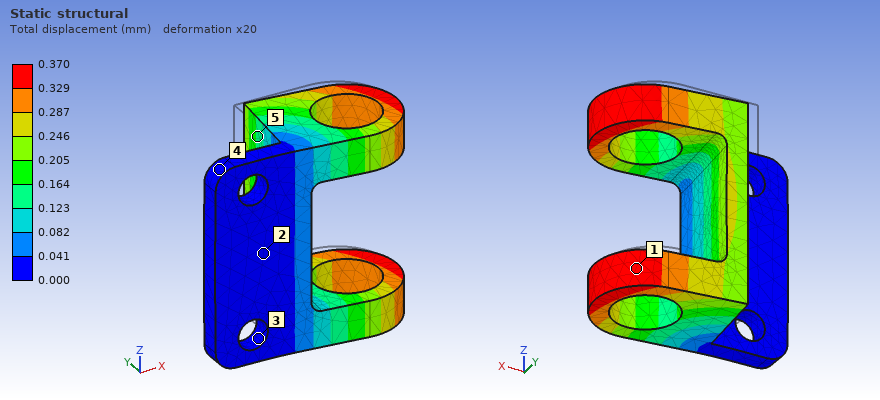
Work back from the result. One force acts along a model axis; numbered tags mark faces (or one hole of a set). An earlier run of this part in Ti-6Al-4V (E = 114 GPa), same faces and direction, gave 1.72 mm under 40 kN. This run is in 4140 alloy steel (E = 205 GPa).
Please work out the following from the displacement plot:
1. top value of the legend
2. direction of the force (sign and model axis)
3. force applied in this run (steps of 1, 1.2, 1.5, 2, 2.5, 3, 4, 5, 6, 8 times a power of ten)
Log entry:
0.370 mm
+X
15 kN
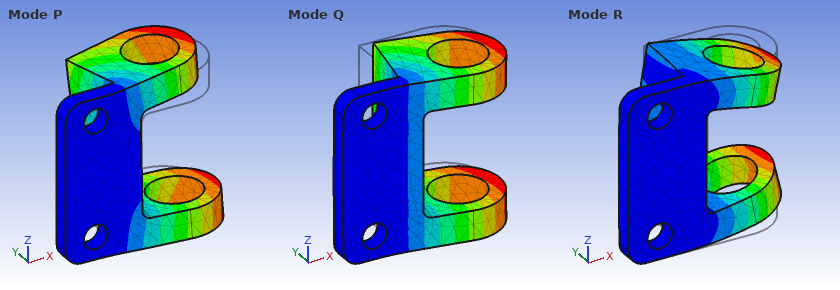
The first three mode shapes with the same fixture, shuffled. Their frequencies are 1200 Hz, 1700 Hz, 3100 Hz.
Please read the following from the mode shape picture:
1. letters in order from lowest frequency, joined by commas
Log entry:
Q, P, R
